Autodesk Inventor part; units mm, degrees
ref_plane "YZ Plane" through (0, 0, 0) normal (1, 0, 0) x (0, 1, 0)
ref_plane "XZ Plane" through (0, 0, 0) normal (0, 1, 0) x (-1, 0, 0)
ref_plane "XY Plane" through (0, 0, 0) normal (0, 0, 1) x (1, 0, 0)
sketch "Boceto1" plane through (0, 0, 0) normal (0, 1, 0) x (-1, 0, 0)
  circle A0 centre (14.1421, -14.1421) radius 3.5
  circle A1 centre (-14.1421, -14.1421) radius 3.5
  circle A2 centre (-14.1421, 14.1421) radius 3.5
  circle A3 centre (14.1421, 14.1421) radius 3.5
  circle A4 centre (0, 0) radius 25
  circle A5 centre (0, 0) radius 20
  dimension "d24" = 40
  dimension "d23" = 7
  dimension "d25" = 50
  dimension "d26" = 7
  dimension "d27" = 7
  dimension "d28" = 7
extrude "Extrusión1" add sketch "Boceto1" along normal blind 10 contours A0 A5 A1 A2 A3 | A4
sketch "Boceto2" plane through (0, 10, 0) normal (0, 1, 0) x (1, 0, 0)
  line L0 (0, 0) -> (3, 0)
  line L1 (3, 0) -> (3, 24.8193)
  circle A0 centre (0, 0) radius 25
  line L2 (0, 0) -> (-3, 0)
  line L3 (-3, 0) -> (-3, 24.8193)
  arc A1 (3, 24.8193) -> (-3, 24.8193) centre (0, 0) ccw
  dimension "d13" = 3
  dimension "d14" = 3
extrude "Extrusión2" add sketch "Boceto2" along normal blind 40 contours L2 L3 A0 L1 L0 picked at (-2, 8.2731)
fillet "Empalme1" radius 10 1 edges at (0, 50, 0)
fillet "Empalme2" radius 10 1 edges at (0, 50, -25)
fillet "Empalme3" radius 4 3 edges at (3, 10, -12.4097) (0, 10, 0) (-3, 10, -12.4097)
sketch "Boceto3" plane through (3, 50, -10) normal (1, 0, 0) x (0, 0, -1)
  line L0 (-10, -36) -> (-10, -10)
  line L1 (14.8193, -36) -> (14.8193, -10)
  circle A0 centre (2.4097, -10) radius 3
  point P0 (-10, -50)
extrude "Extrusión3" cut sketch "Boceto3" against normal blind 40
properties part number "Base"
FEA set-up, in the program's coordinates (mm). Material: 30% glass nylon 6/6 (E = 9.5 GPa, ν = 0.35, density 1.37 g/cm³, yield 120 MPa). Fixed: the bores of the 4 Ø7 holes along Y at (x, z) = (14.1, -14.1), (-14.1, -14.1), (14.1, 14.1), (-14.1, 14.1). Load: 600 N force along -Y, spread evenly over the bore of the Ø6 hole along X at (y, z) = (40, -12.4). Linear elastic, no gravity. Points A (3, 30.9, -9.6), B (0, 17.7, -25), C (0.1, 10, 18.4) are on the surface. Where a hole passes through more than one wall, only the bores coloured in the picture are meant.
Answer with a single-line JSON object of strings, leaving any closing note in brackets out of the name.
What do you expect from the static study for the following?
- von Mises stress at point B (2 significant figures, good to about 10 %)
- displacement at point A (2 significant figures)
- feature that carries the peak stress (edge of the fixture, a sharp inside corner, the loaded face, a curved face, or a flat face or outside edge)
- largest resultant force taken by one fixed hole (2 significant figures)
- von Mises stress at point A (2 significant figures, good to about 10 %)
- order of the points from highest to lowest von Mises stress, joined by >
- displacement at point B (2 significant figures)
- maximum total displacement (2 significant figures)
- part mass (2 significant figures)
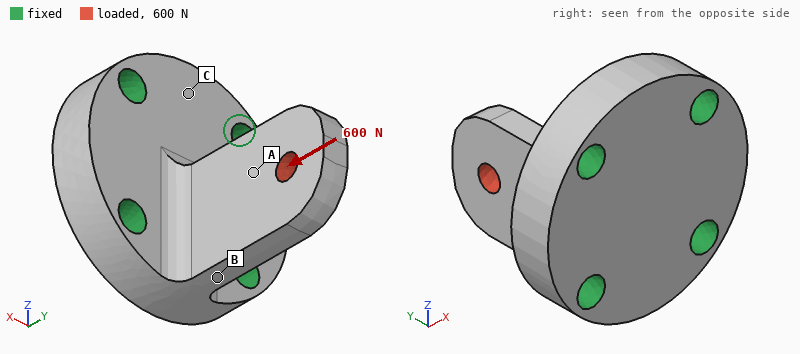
{"von Mises stress at point B": "3.7 MPa", "displacement at point A": "15 µm", "feature that carries the peak stress": "the loaded face", "largest resultant force taken by one fixed hole": "270 N", "von Mises stress at point A": "5.2 MPa", "order of the points from highest to lowest von Mises stress, joined by >": "A > B > C", "displacement at point B": "12 µm", "maximum total displacement": "25 µm", "part mass": "33 g"}
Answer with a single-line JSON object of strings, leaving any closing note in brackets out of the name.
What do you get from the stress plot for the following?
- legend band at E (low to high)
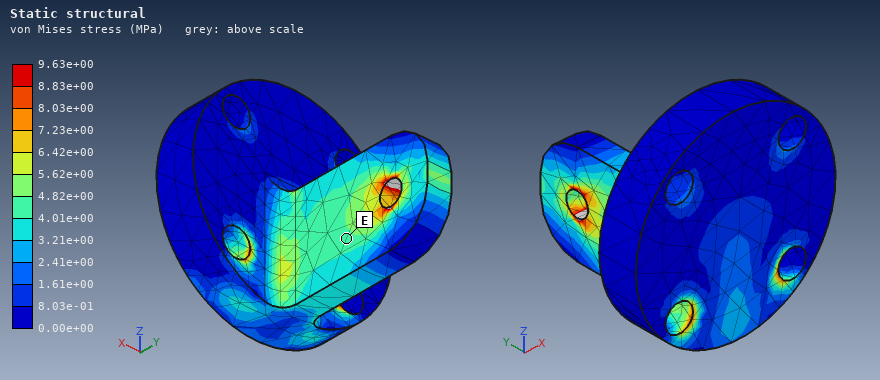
{"legend band at E": "4.01e+00 to 4.82e+00 MPa"}
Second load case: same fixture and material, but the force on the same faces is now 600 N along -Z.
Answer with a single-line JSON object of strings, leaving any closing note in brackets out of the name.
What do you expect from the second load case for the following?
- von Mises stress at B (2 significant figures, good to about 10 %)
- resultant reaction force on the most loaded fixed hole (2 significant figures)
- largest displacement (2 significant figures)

{"von Mises stress at B": "20 MPa", "resultant reaction force on the most loaded fixed hole": "340 N", "largest displacement": "0.24 mm"}
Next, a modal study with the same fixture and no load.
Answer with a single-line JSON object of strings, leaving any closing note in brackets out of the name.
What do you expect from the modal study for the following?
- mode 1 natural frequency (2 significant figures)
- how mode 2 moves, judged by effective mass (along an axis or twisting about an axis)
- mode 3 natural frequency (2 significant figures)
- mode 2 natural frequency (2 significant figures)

{"mode 1 natural frequency": "1800 Hz", "how mode 2 moves, judged by effective mass": "along Z", "mode 3 natural frequency": "5500 Hz", "mode 2 natural frequency": "4400 Hz"}
